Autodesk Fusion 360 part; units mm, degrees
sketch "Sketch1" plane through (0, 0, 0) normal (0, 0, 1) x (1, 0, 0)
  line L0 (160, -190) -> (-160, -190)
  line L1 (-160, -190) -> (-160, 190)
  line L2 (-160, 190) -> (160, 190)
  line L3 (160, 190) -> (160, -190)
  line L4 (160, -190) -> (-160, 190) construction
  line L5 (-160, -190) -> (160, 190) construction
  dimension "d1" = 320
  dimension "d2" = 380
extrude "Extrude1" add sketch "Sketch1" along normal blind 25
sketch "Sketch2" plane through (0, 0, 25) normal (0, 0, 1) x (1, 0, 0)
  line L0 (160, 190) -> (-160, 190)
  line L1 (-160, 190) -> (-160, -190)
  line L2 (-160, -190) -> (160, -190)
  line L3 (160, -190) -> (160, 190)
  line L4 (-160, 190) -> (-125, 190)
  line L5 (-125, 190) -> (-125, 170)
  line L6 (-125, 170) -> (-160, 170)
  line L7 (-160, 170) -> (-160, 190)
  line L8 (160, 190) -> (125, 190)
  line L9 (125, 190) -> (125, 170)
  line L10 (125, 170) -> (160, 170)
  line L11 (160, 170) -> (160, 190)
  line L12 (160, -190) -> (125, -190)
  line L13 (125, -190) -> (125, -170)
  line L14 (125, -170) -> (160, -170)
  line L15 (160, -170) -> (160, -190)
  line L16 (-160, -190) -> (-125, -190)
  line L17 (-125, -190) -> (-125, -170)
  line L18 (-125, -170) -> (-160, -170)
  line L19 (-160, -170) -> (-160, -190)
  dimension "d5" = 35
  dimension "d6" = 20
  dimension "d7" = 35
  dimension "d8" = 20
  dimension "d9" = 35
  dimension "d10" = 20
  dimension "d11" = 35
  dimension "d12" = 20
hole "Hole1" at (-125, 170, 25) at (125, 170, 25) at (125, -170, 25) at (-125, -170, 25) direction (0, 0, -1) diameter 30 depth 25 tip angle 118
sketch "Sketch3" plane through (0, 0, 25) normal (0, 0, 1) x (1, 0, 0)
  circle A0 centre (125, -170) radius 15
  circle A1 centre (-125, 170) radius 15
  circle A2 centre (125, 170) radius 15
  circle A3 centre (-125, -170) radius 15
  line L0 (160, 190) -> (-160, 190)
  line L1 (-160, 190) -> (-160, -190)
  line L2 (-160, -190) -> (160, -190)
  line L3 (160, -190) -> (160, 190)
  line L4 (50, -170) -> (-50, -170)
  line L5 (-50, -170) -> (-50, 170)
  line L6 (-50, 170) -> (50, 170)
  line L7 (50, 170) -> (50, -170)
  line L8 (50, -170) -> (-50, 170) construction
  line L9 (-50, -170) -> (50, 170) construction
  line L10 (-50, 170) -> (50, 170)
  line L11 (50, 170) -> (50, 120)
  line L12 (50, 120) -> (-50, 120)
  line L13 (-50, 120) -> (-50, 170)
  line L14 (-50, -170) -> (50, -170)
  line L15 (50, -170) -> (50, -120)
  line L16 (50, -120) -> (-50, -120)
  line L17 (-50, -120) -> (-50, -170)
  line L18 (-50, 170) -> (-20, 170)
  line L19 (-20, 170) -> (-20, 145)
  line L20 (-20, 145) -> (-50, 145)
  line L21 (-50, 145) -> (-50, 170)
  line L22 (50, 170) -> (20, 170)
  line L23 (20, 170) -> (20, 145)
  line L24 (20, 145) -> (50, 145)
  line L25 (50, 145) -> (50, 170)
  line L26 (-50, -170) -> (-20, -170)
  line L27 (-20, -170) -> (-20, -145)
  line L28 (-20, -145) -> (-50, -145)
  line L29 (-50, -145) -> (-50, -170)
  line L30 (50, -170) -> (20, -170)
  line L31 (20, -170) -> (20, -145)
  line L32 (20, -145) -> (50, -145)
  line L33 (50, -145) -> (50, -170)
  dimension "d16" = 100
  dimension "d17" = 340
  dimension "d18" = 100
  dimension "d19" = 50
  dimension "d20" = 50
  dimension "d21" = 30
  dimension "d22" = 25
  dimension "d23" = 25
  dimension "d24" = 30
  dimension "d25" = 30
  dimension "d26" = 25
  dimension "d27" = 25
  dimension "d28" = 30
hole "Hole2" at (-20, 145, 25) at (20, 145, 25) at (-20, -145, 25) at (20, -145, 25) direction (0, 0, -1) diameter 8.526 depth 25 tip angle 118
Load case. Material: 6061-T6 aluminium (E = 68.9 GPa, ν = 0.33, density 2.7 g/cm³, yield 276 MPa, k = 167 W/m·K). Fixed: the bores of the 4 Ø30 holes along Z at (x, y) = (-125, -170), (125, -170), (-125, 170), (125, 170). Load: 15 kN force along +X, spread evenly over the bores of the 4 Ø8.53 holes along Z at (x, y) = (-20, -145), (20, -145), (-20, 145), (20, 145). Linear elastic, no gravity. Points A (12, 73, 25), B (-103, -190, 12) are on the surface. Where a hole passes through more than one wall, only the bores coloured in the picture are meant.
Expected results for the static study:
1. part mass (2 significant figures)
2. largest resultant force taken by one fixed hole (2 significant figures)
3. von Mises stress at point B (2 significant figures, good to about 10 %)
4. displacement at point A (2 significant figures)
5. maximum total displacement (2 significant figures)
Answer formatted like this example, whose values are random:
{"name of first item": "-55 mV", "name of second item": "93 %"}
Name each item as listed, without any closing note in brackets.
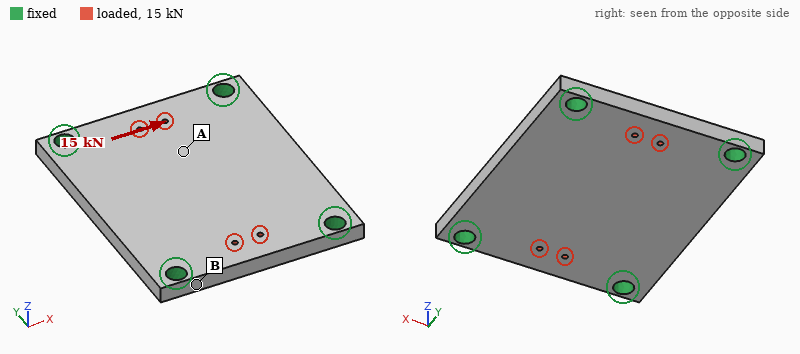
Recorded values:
{"part mass": "8.0 kg", "largest resultant force taken by one fixed hole": "3.8 kN", "von Mises stress at point B": "1.7 MPa", "displacement at point A": "2.2 µm", "maximum total displacement": "4.4 µm"}
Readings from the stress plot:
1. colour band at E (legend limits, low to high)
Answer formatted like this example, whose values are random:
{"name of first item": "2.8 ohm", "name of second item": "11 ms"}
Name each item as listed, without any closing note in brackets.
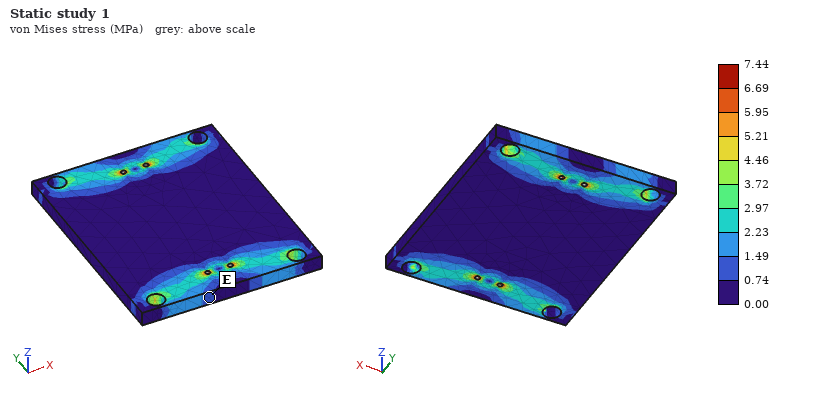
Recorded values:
{"colour band at E": "0.74 to 1.49 MPa"}
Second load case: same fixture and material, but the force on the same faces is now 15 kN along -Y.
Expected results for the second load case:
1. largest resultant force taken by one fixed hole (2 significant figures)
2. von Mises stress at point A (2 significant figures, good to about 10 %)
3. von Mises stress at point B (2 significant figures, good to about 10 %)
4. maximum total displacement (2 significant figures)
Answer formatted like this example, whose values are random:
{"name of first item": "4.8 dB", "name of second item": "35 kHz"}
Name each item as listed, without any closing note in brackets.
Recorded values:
{"largest resultant force taken by one fixed hole": "4.0 kN", "von Mises stress at point A": "1.4 MPa", "von Mises stress at point B": "2.5 MPa", "maximum total displacement": "6.9 µm"}
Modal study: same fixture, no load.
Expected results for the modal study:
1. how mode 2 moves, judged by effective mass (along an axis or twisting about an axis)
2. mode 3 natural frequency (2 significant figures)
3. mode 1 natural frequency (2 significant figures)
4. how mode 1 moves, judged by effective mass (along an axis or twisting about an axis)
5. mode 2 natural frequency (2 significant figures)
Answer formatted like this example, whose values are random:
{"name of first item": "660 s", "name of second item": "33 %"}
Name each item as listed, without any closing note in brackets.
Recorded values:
{"how mode 2 moves, judged by effective mass": "twisting about Y", "mode 3 natural frequency": "1900 Hz", "mode 1 natural frequency": "960 Hz", "how mode 1 moves, judged by effective mass": "along Z", "mode 2 natural frequency": "1400 Hz"}
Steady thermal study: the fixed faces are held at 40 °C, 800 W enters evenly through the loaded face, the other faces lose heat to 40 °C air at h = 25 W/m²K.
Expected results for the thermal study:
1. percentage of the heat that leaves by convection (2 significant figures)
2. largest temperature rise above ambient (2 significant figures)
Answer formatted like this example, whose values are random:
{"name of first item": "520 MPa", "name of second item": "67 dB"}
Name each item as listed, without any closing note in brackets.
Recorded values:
{"percentage of the heat that leaves by convection": "17 %", "largest temperature rise above ambient": "56 K"}
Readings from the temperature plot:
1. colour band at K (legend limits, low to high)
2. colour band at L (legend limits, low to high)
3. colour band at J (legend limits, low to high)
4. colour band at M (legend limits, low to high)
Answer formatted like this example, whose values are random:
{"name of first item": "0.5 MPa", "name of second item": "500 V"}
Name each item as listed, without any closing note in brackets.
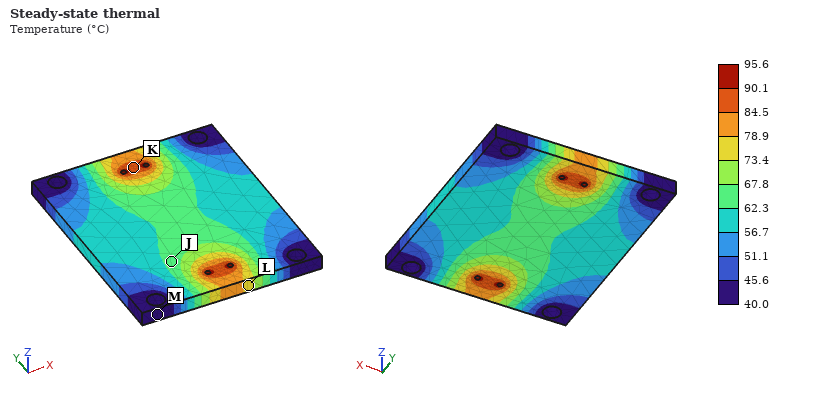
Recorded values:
{"colour band at K": "84.5 to 90.1 °C", "colour band at L": "73.4 to 78.9 °C", "colour band at J": "62.3 to 67.8 °C", "colour band at M": "40.0 to 45.6 °C"}
